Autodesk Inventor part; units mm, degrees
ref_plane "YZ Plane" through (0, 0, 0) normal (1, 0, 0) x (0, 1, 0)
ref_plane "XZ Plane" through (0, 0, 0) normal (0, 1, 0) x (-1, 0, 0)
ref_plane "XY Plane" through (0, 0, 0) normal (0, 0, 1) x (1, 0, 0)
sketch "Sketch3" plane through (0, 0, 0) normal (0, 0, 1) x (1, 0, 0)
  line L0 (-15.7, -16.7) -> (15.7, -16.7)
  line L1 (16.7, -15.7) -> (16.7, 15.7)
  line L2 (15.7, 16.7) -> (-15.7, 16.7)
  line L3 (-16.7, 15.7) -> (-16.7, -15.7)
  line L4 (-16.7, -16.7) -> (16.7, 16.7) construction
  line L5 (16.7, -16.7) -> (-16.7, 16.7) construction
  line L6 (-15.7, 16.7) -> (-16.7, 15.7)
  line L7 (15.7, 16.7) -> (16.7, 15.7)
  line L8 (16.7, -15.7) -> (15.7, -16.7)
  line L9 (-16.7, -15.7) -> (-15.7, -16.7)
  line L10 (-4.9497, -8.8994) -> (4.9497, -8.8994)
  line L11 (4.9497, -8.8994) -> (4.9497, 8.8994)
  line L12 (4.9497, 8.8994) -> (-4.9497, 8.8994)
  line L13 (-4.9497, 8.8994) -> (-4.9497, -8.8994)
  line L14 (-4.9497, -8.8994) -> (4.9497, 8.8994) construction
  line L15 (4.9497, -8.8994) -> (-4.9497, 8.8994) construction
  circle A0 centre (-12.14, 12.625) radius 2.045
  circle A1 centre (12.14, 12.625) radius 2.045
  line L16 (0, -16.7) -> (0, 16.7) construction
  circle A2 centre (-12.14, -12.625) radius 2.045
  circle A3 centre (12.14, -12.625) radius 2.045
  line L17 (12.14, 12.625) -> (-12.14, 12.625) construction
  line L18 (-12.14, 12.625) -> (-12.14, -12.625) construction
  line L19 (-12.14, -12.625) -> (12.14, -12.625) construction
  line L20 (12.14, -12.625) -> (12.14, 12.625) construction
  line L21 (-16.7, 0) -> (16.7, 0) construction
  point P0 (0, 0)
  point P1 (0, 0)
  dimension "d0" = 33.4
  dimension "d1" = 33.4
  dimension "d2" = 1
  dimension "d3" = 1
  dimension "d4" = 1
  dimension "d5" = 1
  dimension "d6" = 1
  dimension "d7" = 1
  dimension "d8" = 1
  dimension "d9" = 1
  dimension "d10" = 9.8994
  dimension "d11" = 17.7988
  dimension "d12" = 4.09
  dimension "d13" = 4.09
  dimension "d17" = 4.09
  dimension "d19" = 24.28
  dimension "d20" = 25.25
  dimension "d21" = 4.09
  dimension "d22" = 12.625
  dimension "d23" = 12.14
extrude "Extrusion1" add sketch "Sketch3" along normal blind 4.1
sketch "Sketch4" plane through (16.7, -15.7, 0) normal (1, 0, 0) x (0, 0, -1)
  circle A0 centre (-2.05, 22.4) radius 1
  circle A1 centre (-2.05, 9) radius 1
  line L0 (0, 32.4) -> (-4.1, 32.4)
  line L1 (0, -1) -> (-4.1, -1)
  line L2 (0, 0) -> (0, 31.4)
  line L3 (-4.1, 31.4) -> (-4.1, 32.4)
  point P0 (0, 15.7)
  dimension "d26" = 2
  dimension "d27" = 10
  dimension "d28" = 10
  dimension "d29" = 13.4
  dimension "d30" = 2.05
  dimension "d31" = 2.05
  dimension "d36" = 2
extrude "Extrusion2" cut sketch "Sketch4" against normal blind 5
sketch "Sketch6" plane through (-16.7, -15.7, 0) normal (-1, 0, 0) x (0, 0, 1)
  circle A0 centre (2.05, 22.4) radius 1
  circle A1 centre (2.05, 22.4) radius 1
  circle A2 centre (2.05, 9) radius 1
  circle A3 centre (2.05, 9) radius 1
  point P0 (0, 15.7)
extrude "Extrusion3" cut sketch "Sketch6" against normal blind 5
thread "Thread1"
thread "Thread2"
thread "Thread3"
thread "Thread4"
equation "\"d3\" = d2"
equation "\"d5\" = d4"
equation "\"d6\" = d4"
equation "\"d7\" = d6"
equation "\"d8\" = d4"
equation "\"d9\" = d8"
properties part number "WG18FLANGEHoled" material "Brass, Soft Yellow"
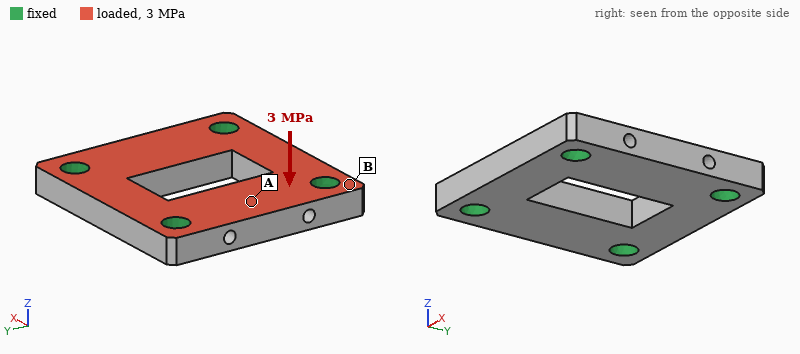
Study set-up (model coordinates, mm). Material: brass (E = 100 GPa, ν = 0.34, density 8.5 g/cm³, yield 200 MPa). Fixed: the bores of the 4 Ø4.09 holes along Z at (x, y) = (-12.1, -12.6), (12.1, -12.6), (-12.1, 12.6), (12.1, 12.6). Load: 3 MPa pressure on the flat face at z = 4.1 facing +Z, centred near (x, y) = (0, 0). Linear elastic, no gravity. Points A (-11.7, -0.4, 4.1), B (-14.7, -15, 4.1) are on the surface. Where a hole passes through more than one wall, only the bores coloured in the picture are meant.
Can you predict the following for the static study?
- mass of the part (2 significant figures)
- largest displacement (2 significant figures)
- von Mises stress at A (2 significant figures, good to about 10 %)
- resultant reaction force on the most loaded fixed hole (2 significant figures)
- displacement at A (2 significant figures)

30 g
8.8 µm
23 MPa
660 N
6.1 µm
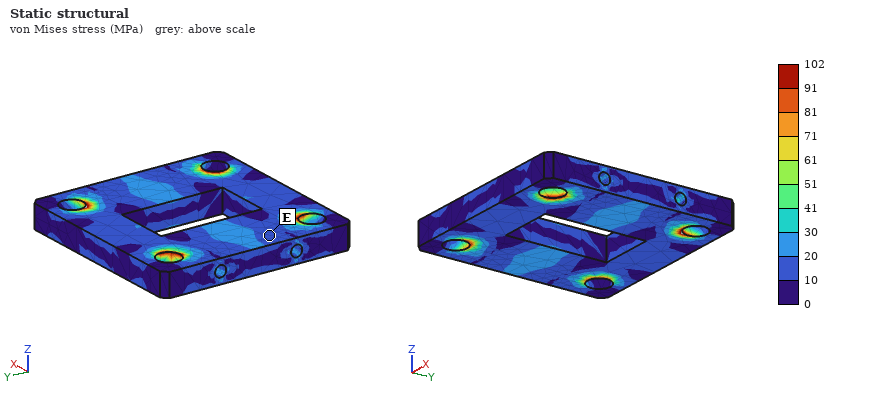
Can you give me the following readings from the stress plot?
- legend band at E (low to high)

10 to 20 MPa
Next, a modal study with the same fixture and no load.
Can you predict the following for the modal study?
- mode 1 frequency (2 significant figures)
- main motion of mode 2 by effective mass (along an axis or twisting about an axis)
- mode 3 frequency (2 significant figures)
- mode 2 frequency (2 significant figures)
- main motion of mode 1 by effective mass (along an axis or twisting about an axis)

20 kHz
twisting about Y
25 kHz
22 kHz
along Z
